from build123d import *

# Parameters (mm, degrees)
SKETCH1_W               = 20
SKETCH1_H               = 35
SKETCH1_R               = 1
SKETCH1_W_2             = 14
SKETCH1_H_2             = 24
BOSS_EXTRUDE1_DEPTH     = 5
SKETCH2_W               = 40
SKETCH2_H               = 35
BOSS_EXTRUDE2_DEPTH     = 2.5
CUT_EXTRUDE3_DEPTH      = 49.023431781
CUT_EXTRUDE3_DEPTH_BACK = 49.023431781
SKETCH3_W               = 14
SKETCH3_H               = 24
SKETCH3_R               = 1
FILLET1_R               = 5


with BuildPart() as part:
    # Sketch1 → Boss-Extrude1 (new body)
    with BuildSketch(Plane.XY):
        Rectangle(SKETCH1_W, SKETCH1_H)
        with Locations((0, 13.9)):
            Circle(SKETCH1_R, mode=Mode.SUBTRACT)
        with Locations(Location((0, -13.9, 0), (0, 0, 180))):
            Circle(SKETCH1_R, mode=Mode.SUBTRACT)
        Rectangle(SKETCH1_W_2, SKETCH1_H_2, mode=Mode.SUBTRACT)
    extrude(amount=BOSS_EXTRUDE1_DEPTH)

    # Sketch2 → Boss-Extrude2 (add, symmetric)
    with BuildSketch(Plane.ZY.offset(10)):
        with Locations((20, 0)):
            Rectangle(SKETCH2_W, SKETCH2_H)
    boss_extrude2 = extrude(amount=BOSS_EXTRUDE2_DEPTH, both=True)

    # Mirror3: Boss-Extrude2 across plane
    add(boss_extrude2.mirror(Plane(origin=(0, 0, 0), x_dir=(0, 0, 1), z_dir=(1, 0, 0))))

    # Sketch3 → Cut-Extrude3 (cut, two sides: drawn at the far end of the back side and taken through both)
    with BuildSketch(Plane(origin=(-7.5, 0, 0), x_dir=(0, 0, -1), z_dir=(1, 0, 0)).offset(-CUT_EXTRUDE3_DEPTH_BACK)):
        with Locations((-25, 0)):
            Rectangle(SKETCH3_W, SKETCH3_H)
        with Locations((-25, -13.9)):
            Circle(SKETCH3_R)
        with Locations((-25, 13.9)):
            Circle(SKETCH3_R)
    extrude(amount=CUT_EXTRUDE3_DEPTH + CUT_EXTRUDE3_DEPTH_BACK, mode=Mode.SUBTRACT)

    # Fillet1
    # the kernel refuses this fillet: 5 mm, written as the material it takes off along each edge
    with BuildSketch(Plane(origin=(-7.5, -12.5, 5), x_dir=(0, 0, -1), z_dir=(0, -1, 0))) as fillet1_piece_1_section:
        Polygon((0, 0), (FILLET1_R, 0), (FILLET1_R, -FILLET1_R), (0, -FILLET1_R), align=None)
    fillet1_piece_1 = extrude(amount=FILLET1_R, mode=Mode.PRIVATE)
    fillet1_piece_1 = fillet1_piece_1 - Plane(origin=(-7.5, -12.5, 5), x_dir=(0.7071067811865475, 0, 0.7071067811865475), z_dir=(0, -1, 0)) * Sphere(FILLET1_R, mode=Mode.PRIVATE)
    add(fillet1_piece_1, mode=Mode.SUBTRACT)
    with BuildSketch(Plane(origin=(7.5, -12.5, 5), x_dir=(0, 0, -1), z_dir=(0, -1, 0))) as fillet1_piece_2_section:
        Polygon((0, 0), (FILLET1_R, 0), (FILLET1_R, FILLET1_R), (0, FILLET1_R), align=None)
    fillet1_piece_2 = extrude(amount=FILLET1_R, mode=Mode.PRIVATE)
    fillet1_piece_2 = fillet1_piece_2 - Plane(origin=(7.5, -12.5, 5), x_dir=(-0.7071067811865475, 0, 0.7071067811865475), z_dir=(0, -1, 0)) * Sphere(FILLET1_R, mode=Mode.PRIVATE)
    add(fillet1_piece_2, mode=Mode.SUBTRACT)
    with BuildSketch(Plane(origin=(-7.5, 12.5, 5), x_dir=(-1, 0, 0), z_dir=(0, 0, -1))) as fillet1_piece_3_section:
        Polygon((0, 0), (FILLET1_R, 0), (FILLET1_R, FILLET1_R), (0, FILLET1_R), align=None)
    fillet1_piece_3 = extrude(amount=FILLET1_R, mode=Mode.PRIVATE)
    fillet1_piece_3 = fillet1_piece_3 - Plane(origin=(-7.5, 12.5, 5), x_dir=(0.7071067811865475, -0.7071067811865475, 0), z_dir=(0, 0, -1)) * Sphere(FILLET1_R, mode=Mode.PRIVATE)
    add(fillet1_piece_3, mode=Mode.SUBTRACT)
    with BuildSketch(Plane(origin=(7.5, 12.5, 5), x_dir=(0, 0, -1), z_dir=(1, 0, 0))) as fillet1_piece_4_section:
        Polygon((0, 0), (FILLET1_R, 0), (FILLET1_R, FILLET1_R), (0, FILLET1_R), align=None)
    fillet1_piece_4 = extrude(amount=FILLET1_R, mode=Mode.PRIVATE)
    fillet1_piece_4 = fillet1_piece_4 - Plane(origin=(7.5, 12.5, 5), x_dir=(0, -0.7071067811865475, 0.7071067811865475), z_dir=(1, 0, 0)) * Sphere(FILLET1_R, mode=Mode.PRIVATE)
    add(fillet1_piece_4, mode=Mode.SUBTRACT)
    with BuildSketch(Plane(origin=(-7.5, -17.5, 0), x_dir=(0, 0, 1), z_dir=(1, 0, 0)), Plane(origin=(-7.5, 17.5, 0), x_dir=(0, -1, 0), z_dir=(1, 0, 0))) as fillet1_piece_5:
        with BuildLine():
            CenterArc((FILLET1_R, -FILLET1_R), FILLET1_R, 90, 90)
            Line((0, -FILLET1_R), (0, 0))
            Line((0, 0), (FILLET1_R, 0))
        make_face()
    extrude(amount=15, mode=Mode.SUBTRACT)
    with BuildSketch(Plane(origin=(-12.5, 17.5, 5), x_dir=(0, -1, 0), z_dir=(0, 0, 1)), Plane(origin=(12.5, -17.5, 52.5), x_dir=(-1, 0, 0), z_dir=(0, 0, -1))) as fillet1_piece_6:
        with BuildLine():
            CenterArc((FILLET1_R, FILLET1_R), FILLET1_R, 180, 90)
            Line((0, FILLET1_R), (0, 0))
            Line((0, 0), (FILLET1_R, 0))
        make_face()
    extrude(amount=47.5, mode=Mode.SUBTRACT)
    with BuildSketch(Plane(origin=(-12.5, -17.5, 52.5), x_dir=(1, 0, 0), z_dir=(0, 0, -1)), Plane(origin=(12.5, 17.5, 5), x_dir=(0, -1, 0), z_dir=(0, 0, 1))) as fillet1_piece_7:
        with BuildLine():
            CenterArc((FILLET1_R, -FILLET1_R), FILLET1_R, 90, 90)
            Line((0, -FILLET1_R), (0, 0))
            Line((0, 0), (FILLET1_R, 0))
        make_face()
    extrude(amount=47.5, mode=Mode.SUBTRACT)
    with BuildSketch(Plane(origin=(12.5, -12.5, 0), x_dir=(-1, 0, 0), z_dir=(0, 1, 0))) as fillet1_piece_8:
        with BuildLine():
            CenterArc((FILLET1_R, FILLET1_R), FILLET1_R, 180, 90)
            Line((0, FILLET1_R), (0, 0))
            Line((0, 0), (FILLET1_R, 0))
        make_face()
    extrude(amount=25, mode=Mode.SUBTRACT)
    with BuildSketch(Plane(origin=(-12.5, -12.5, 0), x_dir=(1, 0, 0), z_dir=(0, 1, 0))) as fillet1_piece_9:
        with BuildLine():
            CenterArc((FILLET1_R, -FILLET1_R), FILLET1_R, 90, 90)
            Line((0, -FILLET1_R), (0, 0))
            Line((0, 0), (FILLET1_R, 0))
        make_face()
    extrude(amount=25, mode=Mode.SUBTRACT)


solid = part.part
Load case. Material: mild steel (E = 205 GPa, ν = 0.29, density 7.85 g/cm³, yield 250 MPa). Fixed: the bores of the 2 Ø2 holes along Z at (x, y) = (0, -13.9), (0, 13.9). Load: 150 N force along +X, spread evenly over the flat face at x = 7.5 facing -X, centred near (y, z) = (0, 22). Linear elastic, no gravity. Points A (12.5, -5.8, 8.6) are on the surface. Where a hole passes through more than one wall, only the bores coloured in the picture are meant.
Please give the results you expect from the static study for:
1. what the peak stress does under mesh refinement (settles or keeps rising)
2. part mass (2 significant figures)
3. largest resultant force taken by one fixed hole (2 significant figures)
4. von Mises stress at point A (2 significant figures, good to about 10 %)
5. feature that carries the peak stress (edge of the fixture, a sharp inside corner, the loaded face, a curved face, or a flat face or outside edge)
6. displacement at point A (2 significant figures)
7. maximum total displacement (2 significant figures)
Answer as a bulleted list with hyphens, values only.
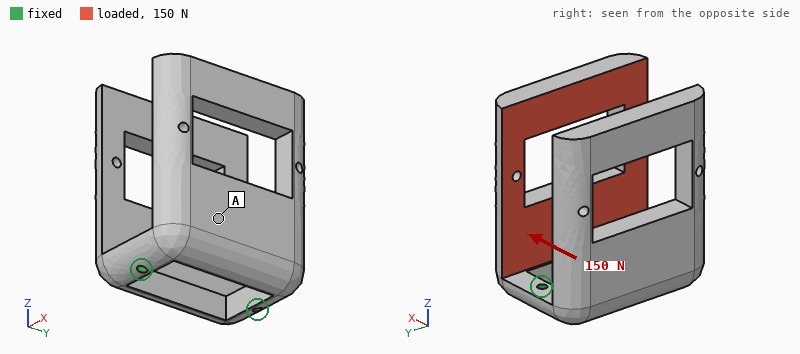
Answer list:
- keeps rising
- 79 g
- 90 N
- 13 MPa
- edge of the fixture
- 17 µm
- 93 µm
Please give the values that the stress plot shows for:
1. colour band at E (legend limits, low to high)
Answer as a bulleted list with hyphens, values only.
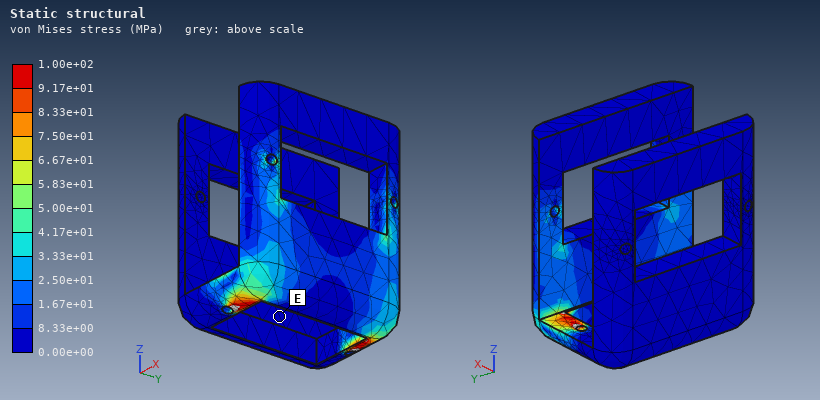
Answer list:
- 0.00e+00 to 8.33e+00 MPa
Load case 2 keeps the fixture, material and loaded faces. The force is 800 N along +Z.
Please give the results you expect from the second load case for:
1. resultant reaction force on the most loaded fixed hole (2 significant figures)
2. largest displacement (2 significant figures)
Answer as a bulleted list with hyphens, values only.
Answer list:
- 400 N
- 25 µm
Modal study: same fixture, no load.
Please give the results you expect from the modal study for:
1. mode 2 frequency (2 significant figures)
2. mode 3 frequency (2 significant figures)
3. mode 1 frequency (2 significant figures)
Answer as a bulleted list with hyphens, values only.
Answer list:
- 1400 Hz
- 3900 Hz
- 1300 Hz
